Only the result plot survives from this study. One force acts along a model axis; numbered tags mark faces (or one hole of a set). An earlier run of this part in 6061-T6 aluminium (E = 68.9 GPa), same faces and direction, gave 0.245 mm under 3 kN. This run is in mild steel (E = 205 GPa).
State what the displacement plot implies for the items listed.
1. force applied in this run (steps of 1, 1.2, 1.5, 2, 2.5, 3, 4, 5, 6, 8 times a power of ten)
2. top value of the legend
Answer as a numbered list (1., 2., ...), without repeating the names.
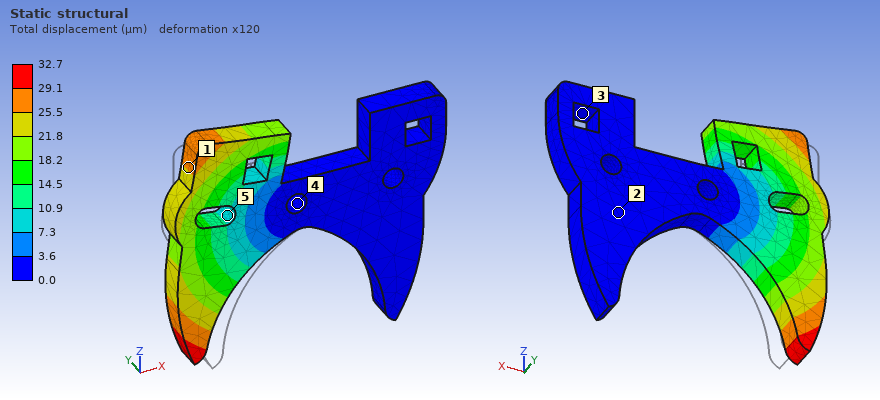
1. 1.2 kN
2. 32.7 µm
